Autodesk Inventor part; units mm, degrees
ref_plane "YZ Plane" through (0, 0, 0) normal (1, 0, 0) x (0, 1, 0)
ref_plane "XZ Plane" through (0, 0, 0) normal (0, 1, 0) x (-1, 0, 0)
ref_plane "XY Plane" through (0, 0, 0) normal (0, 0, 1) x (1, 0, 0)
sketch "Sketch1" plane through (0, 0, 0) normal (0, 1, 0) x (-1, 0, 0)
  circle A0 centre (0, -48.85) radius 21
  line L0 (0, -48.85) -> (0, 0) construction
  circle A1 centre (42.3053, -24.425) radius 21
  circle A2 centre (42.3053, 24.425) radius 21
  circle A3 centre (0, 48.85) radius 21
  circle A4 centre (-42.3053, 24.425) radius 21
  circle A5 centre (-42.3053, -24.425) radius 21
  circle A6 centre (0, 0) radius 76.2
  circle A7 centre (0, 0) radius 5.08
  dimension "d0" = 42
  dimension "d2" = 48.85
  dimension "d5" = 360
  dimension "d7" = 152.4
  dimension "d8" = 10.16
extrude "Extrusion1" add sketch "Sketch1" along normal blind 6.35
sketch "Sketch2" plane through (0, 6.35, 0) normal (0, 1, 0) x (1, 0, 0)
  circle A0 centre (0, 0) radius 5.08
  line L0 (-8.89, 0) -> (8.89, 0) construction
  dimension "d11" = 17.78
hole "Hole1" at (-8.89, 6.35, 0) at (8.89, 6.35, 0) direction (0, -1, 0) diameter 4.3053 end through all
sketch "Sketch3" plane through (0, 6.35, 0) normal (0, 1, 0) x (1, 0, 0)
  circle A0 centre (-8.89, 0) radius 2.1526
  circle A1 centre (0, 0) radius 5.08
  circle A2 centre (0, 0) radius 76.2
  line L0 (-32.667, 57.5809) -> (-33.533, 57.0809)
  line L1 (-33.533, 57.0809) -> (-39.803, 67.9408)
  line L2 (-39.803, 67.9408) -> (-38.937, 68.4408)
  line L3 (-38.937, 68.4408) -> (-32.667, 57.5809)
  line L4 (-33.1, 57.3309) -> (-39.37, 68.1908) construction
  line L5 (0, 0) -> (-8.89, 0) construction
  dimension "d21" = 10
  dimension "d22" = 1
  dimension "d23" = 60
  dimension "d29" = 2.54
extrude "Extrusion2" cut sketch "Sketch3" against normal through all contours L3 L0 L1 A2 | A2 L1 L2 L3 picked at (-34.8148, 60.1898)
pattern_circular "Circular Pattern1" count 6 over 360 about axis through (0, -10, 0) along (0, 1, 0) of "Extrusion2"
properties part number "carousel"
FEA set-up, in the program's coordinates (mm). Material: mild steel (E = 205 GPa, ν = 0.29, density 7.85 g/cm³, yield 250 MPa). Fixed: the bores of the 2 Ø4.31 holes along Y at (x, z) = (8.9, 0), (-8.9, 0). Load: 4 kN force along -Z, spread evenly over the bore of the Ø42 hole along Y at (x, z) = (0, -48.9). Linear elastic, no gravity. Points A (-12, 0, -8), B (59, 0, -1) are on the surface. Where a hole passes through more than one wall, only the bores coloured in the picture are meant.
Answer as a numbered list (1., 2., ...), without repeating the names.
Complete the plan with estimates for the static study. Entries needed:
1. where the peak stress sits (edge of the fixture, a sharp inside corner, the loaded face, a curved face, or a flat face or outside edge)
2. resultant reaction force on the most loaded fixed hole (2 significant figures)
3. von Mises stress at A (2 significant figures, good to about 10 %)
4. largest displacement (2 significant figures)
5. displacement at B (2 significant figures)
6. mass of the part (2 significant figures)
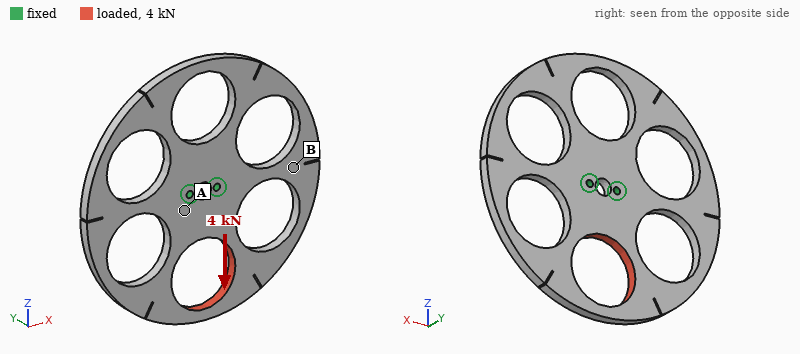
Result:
1. the loaded face
2. 2.0 kN
3. 21 MPa
4. 23 µm
5. 3.7 µm
6. 490 g
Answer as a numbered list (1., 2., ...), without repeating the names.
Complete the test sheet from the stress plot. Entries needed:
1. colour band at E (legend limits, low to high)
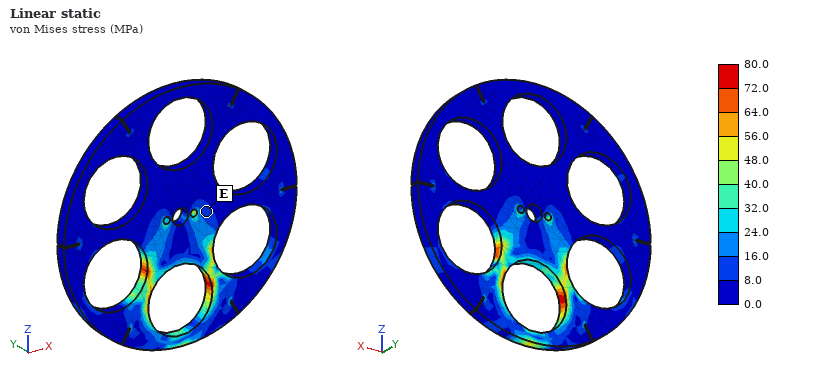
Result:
1. 8.0 to 16.0 MPa
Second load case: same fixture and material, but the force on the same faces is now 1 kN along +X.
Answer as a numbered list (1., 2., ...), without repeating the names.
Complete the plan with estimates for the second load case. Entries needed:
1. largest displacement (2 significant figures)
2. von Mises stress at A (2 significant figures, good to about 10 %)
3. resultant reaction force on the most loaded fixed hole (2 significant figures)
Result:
1. 26 µm
2. 9.8 MPa
3. 2.3 kN
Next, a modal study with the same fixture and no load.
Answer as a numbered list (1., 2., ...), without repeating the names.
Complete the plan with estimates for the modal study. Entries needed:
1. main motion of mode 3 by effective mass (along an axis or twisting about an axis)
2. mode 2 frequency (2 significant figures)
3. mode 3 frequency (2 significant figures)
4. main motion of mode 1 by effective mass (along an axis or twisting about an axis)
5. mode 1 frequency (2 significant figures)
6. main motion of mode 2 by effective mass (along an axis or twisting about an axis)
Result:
1. along Y
2. 810 Hz
3. 850 Hz
4. twisting about X
5. 690 Hz
6. twisting about Z
